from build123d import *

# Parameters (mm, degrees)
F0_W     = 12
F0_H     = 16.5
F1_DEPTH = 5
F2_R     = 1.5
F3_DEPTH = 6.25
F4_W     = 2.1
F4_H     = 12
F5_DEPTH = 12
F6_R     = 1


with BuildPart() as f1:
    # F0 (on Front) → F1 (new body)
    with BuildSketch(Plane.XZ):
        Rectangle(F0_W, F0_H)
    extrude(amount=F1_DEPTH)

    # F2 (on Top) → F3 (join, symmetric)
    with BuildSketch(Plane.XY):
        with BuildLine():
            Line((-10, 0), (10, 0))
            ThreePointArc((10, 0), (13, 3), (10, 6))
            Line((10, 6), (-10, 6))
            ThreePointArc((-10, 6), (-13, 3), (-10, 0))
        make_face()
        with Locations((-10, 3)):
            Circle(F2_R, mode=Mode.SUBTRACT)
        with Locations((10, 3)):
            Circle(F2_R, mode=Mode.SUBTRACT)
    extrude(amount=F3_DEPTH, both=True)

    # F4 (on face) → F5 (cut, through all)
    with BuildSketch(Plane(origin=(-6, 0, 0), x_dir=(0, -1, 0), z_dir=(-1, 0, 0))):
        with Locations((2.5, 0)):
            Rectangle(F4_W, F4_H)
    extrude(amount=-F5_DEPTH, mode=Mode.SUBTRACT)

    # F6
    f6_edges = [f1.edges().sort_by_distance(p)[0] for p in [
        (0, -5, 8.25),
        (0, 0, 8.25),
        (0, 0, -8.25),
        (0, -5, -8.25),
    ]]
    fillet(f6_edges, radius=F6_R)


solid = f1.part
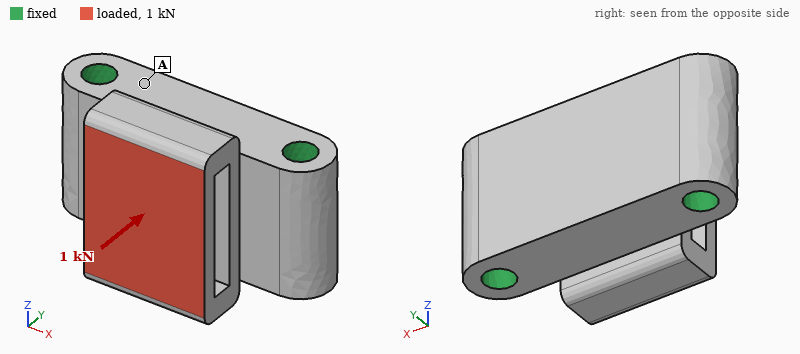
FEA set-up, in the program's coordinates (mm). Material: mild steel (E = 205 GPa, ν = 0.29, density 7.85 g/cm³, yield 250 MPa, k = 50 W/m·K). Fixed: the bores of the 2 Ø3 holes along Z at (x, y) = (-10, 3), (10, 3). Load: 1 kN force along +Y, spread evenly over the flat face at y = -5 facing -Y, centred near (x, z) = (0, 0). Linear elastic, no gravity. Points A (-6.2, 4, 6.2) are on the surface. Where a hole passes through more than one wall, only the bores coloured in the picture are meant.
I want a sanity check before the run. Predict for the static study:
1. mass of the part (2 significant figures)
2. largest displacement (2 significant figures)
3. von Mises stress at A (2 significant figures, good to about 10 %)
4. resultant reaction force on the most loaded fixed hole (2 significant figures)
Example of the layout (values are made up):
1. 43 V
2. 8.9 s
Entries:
1. 18 g
2. 15 µm
3. 20 MPa
4. 530 N
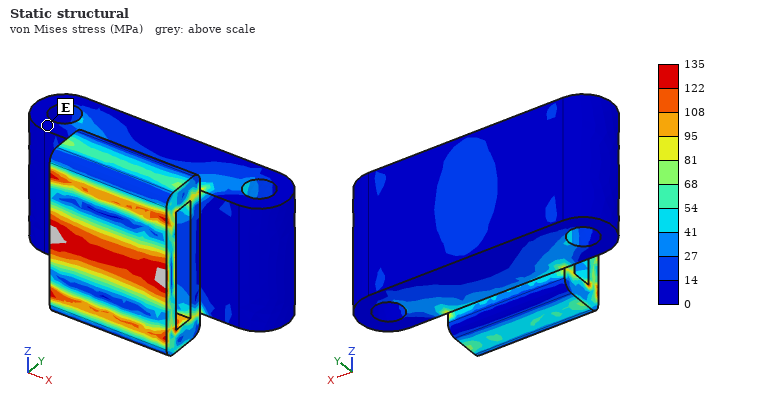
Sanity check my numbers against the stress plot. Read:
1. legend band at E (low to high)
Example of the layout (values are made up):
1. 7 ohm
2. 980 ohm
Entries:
1. 0 to 14 MPa
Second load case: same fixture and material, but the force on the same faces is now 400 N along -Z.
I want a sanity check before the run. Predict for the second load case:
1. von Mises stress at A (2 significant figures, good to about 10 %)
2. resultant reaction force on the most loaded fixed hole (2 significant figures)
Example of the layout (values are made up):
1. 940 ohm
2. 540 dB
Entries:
1. 15 MPa
2. 200 N
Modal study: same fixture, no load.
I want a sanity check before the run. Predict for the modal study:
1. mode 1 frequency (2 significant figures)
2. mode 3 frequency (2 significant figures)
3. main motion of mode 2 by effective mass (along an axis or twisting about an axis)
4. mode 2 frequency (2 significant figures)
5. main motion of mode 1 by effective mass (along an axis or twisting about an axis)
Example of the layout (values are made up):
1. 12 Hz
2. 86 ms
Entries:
1. 26 kHz
2. 41 kHz
3. along Y
4. 33 kHz
5. along Z
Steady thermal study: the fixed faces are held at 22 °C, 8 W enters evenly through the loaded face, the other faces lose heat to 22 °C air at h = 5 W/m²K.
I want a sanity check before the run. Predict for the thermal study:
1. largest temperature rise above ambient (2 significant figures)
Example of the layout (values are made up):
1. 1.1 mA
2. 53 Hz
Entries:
1. 37 K
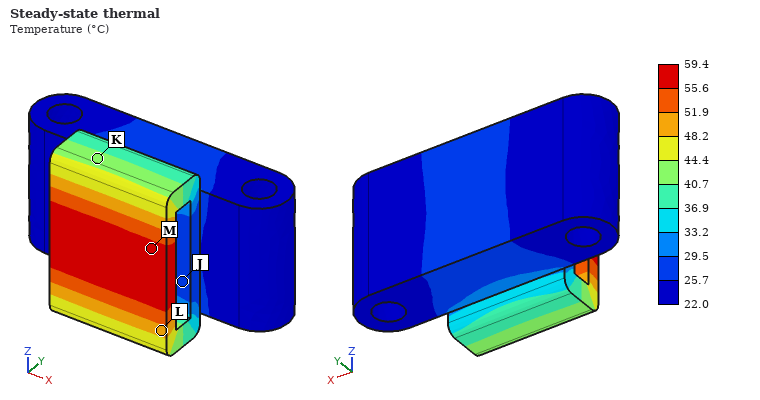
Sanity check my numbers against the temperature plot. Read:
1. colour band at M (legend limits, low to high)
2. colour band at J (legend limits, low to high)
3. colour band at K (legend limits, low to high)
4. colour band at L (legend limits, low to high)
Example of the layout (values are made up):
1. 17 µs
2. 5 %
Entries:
1. 55.6 to 59.4 °C
2. 25.7 to 29.5 °C
3. 40.7 to 44.4 °C
4. 48.2 to 51.9 °C
